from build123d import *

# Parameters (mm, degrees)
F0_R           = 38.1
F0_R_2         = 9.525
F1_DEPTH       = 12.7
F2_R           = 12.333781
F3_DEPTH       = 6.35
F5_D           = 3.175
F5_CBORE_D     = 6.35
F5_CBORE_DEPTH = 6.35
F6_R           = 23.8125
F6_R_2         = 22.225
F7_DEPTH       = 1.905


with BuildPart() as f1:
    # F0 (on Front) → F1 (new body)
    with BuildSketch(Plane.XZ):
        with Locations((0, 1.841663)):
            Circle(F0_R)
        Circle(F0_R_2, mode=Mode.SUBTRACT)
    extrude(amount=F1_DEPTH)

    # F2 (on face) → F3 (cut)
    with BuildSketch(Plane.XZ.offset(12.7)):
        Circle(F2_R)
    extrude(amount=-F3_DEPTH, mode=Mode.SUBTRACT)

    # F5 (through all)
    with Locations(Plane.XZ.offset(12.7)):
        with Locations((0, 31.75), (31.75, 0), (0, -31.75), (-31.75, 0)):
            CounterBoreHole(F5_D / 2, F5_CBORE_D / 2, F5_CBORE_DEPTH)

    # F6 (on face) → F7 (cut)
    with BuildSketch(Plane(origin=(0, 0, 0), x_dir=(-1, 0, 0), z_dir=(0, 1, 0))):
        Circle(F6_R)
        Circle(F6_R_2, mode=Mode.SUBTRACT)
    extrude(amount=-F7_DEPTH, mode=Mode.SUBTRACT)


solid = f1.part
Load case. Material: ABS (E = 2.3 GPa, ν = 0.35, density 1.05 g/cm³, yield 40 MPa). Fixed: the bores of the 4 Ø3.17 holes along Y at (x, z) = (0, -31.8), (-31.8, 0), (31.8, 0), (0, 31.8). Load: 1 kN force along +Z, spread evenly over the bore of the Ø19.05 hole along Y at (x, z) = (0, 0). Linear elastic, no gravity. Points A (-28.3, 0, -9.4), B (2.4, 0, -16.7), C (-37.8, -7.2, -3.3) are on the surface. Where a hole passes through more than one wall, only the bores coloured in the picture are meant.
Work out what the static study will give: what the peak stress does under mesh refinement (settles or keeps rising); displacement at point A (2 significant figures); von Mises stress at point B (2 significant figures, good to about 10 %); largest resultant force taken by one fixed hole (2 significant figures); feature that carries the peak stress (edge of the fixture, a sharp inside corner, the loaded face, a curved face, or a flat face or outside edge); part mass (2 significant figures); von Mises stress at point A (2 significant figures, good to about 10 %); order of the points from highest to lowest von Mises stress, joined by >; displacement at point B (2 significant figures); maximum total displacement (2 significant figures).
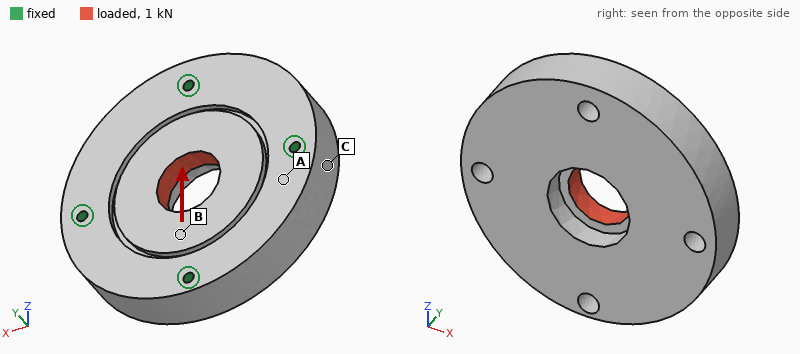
keeps rising
8.7 µm
2.6 MPa
290 N
edge of the fixture
54 g
1.2 MPa
B > A > C
23 µm
33 µm
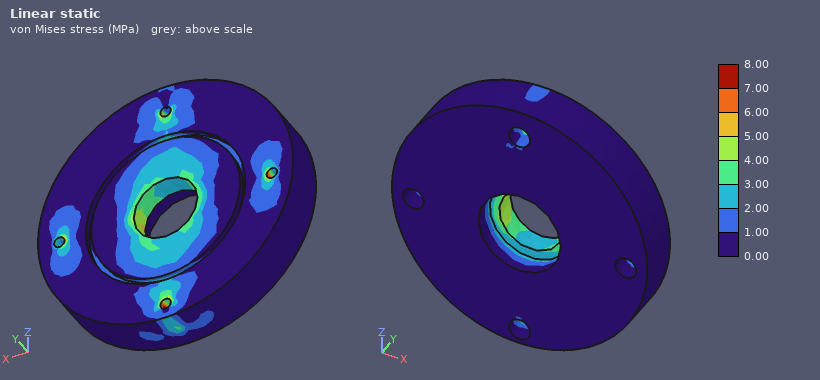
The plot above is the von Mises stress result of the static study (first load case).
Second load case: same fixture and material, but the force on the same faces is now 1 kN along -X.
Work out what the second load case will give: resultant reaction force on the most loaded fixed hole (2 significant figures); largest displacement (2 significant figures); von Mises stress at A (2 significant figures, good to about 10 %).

280 N
33 µm
0.92 MPa
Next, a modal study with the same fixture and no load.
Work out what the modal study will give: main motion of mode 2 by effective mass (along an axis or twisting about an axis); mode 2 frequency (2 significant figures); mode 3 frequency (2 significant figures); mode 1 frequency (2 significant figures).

along Y
3900 Hz
4100 Hz
3500 Hz
